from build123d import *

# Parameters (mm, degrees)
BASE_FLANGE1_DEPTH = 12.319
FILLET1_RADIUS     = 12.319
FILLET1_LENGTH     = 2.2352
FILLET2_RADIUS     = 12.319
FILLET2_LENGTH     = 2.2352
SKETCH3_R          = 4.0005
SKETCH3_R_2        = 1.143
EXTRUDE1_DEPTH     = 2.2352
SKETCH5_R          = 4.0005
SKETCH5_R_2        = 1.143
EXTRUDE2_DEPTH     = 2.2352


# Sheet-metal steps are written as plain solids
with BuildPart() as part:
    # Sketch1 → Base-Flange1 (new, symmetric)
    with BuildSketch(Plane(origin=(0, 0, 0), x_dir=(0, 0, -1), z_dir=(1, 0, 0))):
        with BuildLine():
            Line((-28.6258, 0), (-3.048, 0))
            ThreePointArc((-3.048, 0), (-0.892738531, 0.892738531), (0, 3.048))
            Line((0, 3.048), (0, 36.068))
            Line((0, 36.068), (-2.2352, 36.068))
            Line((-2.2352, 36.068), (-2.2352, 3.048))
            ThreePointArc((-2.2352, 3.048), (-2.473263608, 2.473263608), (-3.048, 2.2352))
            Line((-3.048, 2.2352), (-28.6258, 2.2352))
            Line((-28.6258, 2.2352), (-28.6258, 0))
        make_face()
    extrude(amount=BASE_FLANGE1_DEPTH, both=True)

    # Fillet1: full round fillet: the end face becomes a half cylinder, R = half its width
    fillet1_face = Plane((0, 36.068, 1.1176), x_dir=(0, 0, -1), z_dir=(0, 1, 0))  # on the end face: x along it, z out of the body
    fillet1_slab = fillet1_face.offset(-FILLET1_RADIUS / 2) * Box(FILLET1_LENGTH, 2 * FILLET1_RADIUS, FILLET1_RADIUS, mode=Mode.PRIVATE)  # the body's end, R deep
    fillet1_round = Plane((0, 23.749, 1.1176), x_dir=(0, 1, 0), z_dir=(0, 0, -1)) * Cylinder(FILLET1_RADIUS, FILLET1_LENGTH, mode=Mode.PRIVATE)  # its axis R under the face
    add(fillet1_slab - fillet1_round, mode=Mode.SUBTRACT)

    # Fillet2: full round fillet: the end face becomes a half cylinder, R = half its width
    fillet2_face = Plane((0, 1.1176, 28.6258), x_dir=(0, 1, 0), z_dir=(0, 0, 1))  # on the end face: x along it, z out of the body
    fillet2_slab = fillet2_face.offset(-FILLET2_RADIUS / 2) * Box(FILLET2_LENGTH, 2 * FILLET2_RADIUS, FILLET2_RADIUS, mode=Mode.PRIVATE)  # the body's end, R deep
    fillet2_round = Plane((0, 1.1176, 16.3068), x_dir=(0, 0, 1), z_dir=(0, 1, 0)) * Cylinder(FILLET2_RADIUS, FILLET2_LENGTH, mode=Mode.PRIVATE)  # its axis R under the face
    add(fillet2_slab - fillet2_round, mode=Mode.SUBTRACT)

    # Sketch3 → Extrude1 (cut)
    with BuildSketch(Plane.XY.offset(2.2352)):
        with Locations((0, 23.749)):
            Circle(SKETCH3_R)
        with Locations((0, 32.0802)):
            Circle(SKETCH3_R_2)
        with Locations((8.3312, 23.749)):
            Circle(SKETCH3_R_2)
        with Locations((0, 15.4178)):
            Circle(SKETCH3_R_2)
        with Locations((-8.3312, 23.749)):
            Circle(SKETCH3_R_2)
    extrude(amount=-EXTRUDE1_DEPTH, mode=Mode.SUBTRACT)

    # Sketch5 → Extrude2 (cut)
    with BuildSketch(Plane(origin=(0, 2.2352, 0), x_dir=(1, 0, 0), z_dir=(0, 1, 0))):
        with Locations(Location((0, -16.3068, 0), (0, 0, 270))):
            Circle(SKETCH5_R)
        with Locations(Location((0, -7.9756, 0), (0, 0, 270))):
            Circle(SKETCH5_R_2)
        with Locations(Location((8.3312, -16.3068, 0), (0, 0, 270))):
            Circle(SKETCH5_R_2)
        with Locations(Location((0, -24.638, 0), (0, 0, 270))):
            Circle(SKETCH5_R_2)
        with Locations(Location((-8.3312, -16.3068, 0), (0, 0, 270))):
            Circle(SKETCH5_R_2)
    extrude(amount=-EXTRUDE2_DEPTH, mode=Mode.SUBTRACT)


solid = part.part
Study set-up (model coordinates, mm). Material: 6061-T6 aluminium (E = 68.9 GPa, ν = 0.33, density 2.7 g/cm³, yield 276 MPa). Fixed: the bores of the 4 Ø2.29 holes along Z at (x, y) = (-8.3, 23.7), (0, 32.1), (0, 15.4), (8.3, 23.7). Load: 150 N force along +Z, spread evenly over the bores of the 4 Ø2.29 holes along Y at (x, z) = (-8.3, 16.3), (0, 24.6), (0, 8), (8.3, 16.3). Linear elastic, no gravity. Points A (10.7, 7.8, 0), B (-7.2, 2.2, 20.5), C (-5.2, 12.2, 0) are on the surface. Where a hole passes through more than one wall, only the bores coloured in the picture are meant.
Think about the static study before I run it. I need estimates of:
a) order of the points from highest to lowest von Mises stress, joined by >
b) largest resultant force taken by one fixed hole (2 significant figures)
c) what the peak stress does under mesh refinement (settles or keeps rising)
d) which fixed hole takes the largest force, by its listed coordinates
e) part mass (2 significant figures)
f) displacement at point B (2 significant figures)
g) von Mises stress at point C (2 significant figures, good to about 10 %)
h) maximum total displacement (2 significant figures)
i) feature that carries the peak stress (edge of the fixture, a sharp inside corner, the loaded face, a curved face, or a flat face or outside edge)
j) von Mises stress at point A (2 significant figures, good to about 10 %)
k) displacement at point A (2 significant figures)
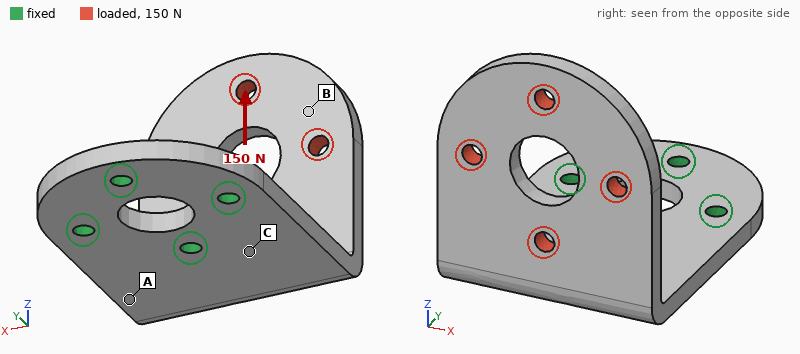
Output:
C > A > B
250 N
keeps rising
(0, 15.4)
7.6 g
0.23 mm
70 MPa
0.31 mm
edge of the fixture
44 MPa
0.049 mm
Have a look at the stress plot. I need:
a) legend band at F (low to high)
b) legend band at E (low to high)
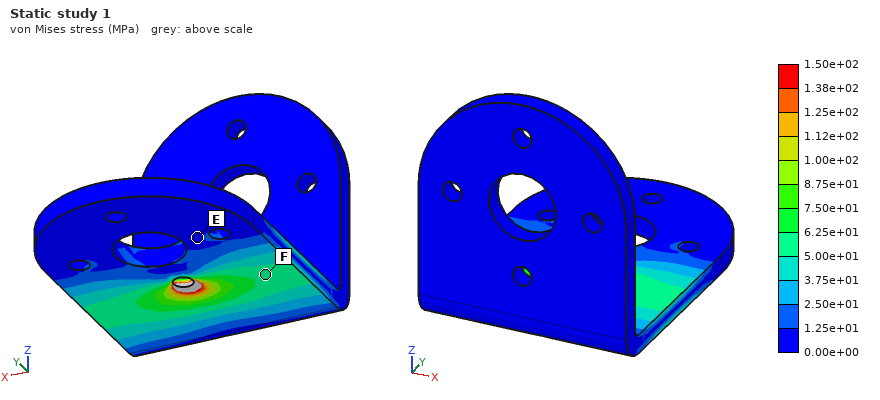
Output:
5.00e+01 to 6.25e+01 MPa
0.00e+00 to 1.25e+01 MPa
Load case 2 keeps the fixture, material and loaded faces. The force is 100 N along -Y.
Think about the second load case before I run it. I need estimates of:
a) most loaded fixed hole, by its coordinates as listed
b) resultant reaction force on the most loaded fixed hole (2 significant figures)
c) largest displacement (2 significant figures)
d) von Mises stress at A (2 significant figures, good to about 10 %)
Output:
(0, 15.4)
120 N
0.56 mm
70 MPa
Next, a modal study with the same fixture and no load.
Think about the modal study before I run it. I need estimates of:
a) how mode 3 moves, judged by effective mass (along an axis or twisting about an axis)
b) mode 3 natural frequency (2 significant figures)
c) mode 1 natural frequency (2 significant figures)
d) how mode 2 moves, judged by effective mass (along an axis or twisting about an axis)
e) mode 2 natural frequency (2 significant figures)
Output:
along Z
4500 Hz
1600 Hz
along X
2300 Hz
